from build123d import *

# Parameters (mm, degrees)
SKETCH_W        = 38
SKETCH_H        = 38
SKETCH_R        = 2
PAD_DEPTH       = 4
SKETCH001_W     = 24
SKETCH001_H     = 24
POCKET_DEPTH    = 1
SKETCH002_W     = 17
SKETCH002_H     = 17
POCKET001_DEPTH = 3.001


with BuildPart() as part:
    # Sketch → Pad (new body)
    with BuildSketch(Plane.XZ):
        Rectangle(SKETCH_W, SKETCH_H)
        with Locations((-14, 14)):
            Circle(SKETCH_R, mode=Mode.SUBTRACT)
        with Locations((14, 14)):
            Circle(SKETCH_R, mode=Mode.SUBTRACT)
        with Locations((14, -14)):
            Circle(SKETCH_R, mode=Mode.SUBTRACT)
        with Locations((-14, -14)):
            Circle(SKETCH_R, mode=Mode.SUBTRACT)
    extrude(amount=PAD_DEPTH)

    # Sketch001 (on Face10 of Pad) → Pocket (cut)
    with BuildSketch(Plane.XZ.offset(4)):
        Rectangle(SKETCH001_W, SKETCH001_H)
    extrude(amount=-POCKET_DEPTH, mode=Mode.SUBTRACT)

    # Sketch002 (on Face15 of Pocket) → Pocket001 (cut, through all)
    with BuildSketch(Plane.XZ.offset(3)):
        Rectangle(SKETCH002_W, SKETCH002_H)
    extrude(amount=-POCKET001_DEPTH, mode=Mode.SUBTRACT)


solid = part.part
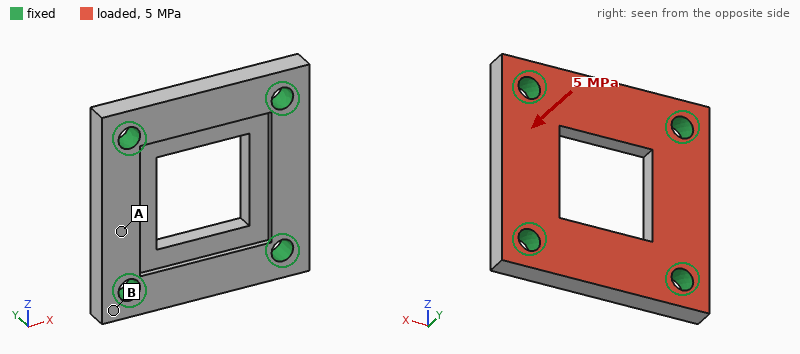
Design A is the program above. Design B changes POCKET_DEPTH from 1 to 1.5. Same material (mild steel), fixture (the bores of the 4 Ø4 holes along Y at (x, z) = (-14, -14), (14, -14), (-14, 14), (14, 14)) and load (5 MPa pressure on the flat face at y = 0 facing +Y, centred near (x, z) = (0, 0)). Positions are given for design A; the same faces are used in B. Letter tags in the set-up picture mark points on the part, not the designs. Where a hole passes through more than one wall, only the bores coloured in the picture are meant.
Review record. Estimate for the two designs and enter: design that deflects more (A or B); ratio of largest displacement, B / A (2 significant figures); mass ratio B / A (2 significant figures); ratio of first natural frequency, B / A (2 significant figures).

B
1.1
0.97
1.00
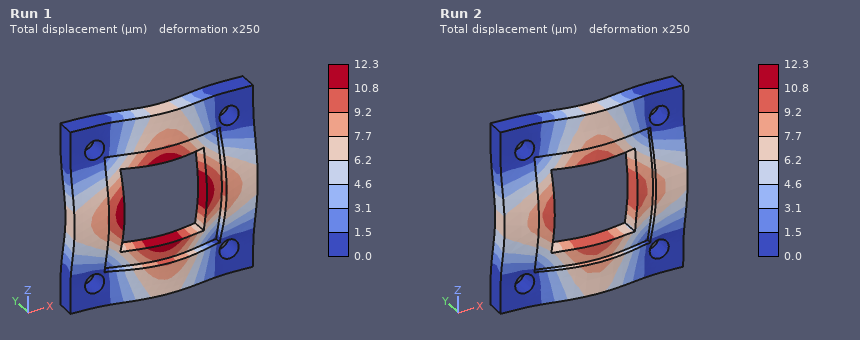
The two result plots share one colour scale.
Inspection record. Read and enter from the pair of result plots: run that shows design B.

Run 1
